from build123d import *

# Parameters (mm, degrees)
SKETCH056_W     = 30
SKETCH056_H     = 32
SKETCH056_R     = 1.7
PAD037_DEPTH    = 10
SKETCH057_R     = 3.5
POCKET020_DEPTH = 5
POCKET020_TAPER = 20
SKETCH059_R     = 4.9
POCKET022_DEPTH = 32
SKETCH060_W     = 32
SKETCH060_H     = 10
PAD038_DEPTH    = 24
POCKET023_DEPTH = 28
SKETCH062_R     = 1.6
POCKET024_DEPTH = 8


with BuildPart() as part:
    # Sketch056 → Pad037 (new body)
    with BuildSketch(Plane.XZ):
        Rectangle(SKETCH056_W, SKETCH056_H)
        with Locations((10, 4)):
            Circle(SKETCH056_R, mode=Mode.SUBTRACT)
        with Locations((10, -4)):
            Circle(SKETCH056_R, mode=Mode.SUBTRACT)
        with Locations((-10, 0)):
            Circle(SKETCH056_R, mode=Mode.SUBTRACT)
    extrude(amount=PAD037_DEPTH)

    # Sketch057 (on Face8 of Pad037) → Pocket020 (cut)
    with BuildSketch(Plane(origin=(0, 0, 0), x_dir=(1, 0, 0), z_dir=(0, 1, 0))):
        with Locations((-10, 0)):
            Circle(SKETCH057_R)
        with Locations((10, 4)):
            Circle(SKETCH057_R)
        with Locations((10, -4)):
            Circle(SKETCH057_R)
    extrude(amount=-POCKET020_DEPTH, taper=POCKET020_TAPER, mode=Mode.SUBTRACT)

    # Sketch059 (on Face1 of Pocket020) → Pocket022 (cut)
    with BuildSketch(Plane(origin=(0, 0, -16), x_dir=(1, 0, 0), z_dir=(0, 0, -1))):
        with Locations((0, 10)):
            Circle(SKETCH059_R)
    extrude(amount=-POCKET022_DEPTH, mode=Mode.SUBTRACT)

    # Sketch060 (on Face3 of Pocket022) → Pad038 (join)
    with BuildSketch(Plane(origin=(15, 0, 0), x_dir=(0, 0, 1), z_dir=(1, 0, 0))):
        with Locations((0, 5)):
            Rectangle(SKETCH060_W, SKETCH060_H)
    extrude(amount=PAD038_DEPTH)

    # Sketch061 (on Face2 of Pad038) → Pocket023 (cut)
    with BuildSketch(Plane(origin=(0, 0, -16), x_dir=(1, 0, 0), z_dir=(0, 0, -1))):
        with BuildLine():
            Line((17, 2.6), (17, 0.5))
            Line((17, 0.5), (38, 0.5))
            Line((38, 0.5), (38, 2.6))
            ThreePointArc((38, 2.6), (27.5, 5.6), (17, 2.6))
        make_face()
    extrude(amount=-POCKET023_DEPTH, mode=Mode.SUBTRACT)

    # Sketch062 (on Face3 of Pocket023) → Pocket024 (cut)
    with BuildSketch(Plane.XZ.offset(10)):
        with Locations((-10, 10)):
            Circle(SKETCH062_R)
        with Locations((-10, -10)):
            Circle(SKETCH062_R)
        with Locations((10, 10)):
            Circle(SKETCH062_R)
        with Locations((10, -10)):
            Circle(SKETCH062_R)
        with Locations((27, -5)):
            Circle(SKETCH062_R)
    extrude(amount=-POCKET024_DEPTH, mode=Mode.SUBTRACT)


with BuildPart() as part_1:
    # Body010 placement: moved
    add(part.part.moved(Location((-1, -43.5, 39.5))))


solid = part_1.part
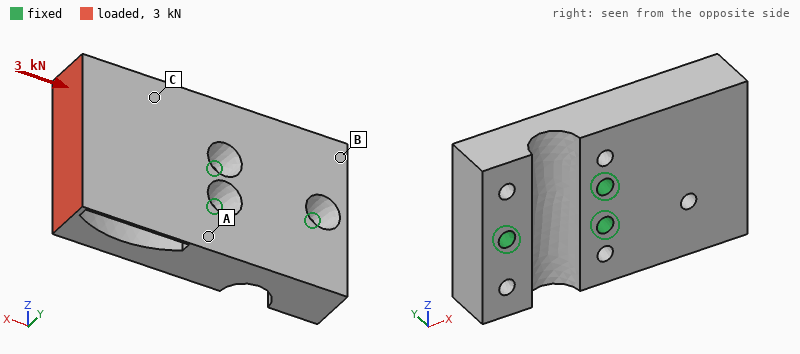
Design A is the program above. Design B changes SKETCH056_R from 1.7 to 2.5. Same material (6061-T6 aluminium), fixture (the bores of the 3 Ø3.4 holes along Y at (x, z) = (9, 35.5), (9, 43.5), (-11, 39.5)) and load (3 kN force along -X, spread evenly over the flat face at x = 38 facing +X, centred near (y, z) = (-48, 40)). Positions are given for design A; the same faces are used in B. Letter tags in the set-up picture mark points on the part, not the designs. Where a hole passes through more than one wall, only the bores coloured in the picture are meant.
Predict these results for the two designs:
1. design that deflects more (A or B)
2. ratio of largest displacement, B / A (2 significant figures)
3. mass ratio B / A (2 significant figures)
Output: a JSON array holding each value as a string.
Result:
["A", "0.87", "0.98"]
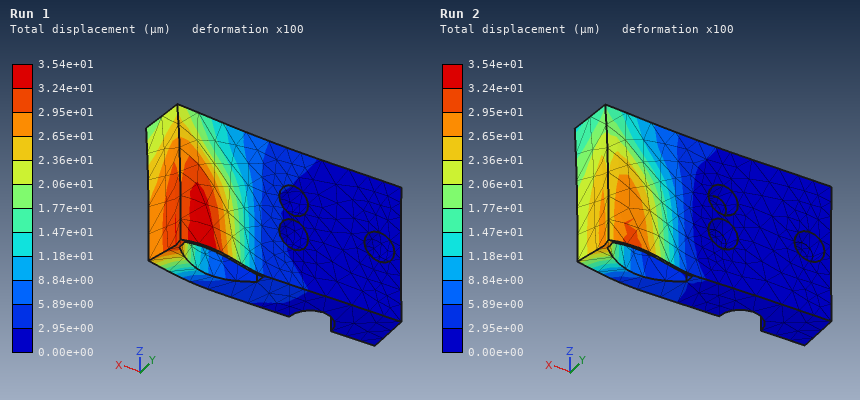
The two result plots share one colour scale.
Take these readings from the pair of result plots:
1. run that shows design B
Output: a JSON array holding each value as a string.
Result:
["Run 2"]
